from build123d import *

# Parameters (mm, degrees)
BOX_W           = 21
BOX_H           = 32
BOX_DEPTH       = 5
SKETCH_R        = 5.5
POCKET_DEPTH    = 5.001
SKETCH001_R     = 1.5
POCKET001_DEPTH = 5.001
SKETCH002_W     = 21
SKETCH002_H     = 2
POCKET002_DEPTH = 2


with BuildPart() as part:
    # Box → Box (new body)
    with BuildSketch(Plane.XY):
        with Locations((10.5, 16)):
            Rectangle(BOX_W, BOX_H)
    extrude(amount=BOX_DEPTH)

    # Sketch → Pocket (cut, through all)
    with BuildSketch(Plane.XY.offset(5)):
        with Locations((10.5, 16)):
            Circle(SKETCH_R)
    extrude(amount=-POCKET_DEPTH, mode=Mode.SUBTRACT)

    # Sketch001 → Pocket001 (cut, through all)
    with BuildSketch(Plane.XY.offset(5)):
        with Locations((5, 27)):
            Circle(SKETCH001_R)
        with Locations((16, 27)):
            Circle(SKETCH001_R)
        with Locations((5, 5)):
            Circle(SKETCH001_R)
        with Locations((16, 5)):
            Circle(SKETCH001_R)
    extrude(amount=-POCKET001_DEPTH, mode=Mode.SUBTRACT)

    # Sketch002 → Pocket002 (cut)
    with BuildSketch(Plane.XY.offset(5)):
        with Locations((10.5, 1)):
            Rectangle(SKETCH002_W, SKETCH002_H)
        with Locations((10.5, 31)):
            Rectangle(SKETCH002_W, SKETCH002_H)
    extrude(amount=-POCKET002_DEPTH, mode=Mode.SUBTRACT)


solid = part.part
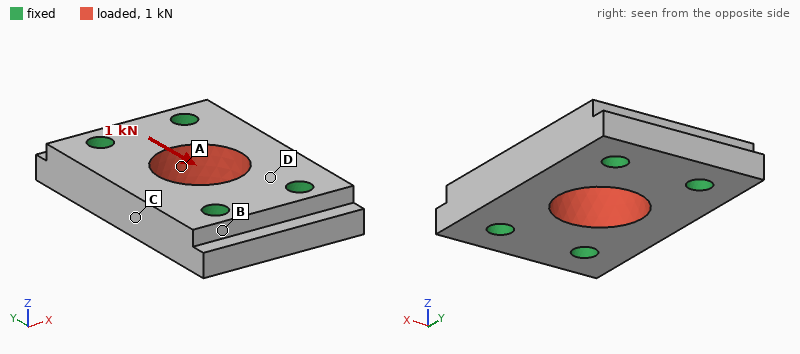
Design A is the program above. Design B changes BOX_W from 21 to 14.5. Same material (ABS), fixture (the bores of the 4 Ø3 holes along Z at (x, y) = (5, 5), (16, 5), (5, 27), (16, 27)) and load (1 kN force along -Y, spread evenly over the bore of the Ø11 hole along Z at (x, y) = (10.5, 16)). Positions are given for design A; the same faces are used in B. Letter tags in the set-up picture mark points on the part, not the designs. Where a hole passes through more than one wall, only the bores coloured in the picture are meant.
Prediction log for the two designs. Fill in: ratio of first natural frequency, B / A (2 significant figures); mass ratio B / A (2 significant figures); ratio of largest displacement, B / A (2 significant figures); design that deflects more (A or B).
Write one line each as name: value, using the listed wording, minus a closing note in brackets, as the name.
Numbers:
ratio of first natural frequency, B / A: 1.2
mass ratio B / A: 0.62
ratio of largest displacement, B / A: 1.3
design that deflects more: B
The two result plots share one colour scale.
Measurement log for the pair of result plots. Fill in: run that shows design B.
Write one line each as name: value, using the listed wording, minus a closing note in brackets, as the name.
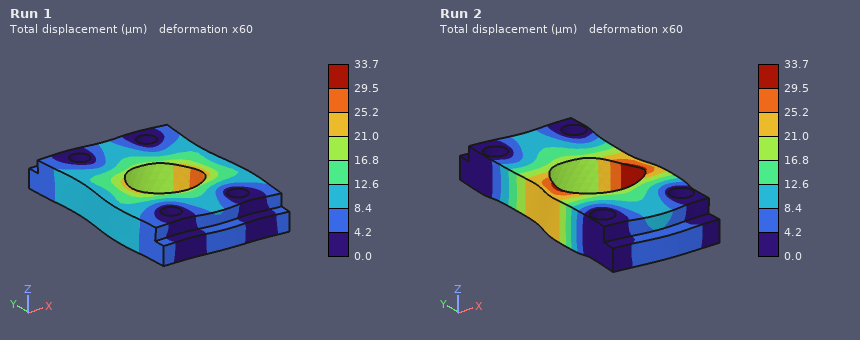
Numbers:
run that shows design B: Run 2
